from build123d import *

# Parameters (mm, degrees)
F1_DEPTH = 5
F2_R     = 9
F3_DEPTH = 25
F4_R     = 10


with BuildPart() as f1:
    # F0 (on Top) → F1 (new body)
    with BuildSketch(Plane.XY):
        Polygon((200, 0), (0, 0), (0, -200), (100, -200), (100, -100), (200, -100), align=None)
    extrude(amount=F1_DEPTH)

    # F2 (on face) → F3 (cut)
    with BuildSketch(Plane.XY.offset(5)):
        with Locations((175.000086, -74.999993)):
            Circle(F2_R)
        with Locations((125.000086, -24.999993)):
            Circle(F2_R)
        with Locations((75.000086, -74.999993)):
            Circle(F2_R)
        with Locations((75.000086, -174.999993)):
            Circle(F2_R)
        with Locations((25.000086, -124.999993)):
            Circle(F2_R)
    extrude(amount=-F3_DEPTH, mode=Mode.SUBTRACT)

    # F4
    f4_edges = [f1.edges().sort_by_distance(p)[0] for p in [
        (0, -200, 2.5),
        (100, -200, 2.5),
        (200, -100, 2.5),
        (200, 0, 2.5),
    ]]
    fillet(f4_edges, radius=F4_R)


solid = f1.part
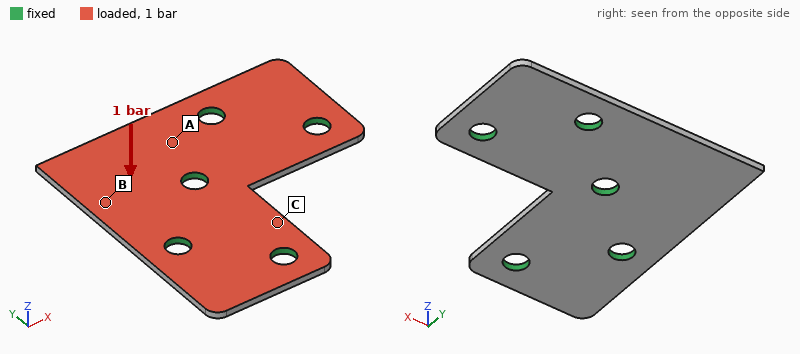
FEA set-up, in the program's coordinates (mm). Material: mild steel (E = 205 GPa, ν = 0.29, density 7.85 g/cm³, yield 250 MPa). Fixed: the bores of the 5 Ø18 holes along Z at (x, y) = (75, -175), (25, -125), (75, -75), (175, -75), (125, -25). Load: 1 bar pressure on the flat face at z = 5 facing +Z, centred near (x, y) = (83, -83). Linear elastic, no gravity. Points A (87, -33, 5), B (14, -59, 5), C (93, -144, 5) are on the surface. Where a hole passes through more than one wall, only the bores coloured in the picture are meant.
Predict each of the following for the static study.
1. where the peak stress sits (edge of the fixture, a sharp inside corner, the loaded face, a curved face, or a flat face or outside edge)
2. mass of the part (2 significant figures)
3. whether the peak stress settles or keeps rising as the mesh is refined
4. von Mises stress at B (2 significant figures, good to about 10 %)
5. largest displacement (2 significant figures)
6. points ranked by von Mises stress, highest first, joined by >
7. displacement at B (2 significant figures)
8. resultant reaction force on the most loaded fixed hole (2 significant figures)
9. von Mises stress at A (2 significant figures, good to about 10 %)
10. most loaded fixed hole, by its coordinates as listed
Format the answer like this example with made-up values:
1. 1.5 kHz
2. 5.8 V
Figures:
1. edge of the fixture
2. 1.1 kg
3. keeps rising
4. 17 MPa
5. 0.25 mm
6. A > B > C
7. 0.088 mm
8. 890 N
9. 28 MPa
10. (75, -75)
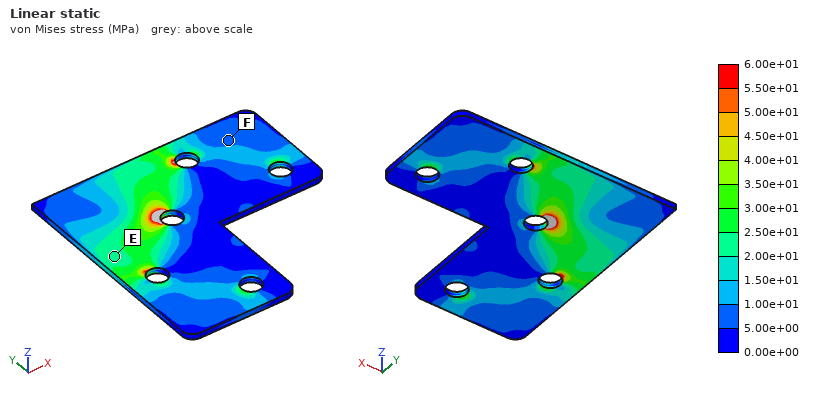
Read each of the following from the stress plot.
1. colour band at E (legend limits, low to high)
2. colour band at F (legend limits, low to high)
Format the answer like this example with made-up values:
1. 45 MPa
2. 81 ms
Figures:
1. 2.00e+01 to 2.50e+01 MPa
2. 5.00e+00 to 1.00e+01 MPa
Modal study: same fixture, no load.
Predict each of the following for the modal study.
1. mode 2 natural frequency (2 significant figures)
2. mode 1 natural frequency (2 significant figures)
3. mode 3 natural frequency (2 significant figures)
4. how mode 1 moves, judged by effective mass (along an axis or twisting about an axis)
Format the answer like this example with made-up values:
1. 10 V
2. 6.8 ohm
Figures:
1. 1700 Hz
2. 730 Hz
3. 1700 Hz
4. along Z
